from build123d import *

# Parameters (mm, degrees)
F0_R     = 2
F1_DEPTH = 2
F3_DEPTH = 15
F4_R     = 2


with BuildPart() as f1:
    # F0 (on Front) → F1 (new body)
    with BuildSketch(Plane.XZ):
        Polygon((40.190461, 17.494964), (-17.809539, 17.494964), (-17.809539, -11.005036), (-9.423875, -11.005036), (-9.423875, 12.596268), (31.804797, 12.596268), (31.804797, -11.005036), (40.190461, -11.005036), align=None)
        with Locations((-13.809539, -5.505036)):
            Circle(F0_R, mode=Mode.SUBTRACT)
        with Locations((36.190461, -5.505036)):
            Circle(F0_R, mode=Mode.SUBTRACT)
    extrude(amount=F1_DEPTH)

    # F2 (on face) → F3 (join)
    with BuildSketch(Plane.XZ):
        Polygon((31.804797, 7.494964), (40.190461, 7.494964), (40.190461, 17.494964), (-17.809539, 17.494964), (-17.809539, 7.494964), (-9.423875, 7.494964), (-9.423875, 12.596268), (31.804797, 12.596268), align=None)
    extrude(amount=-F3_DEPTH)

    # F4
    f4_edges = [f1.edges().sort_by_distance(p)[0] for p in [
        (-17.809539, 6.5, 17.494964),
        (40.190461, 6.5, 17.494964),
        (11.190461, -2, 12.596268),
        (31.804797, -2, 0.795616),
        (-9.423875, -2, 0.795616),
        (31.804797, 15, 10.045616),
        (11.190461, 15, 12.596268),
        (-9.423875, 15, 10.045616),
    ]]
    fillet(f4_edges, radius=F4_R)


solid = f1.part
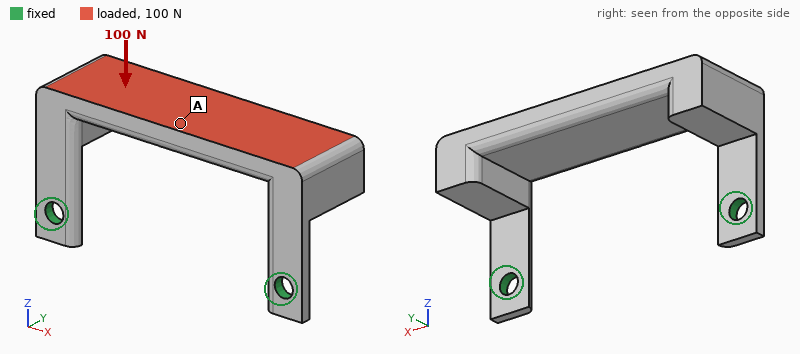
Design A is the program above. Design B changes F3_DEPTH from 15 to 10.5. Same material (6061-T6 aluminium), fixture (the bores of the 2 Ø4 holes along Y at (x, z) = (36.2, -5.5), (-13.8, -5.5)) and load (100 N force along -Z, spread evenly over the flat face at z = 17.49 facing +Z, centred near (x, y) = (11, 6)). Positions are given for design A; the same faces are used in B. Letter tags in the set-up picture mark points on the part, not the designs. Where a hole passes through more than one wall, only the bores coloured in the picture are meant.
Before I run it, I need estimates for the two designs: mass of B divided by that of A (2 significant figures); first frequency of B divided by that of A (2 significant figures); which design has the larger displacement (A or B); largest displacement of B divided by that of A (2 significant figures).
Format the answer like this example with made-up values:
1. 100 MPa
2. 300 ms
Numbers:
1. 0.75
2. 1.3
3. A
4. 0.61
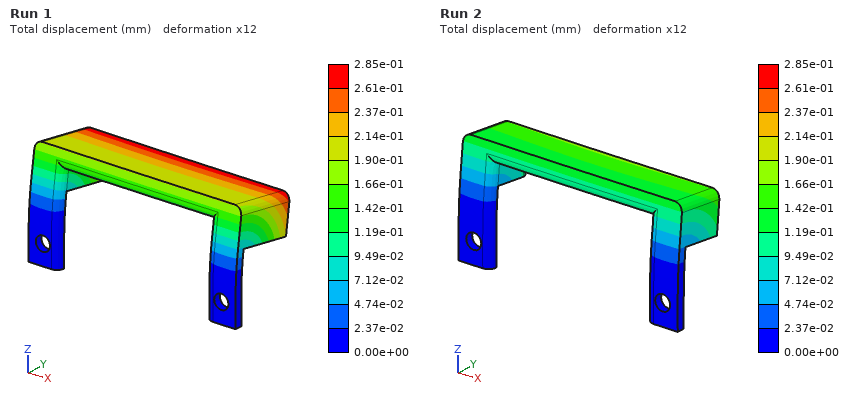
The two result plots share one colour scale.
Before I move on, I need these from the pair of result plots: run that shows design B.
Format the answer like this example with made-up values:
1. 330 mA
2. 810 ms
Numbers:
1. Run 2
